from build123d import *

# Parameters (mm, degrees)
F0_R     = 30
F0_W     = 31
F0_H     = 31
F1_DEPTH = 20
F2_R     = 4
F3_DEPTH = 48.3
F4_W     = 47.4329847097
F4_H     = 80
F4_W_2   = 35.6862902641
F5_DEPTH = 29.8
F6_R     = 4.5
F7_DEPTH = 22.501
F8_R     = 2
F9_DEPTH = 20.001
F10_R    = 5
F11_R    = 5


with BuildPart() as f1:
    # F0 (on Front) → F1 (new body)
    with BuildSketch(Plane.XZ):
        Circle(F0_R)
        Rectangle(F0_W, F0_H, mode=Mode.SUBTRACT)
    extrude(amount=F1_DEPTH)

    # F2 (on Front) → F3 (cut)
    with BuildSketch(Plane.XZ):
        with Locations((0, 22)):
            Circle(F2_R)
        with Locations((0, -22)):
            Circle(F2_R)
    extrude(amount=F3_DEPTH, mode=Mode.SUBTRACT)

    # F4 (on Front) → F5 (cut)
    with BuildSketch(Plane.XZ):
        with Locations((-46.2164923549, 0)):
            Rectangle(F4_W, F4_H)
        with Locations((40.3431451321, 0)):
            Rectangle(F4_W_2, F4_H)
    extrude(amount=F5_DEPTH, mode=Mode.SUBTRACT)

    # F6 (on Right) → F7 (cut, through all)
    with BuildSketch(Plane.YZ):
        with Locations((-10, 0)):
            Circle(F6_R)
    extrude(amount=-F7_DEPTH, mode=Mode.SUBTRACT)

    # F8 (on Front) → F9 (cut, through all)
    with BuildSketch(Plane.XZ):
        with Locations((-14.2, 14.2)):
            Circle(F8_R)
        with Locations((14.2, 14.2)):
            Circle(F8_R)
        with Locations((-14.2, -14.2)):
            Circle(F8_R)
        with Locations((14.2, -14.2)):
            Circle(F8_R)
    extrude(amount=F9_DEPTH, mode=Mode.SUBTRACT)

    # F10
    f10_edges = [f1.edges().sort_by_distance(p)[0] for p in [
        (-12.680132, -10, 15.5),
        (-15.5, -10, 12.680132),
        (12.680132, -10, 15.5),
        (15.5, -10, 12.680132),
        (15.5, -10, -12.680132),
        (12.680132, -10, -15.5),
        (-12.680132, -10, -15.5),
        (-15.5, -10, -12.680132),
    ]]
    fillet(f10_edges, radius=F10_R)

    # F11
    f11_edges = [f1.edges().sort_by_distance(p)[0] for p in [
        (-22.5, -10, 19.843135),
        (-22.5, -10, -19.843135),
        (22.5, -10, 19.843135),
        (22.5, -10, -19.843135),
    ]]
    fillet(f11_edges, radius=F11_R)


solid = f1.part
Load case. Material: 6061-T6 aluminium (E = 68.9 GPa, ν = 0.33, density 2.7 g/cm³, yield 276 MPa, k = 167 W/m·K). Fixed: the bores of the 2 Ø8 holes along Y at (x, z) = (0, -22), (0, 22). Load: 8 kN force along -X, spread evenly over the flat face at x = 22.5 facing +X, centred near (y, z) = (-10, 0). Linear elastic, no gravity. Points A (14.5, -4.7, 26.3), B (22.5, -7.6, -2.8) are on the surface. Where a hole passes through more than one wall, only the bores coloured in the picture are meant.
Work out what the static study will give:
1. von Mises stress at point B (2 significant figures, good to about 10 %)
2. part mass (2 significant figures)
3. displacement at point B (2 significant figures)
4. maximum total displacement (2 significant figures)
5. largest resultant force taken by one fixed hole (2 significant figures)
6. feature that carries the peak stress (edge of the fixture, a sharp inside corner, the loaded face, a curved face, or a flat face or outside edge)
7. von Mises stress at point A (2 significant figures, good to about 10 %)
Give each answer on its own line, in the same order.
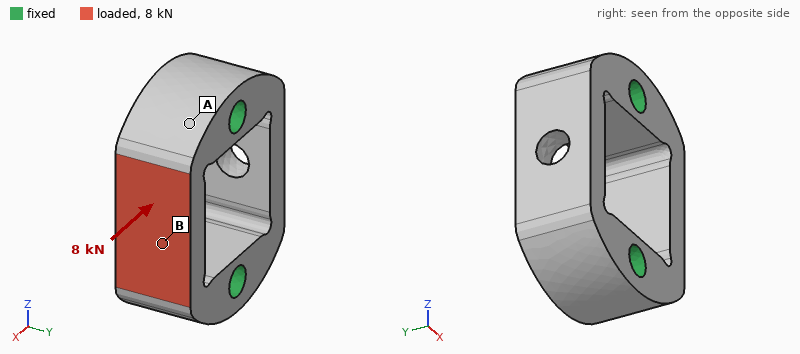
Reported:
100 MPa
71 g
54 µm
61 µm
4.6 kN
a curved face
21 MPa
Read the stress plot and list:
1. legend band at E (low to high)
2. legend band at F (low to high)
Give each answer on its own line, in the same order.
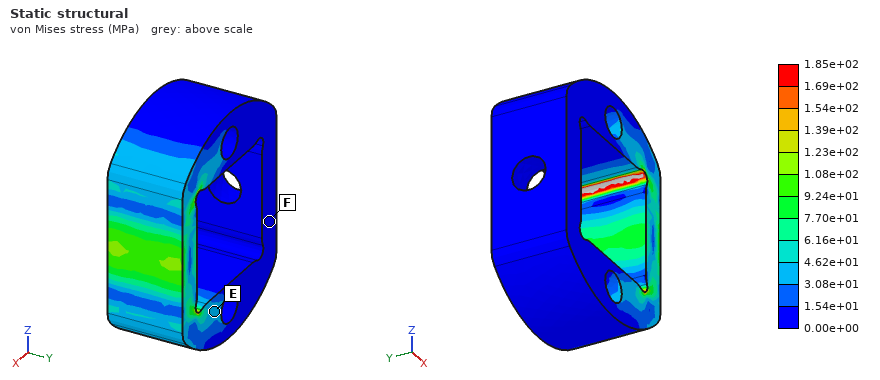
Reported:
3.08e+01 to 4.62e+01 MPa
0.00e+00 to 1.54e+01 MPa
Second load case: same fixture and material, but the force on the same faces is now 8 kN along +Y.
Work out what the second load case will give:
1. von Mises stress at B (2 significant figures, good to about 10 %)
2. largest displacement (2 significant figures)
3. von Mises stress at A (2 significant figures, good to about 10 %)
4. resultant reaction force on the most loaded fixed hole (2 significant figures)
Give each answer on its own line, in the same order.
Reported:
31 MPa
75 µm
23 MPa
4.0 kN
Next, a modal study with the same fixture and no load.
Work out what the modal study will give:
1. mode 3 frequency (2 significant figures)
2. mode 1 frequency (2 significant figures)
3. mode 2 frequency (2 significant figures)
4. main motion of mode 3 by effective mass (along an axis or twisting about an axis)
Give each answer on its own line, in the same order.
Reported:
18 kHz
17 kHz
17 kHz
along Y
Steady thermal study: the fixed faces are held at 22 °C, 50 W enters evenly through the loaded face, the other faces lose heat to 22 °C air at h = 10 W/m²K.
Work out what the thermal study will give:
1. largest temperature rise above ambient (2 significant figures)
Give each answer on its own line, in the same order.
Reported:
22 K
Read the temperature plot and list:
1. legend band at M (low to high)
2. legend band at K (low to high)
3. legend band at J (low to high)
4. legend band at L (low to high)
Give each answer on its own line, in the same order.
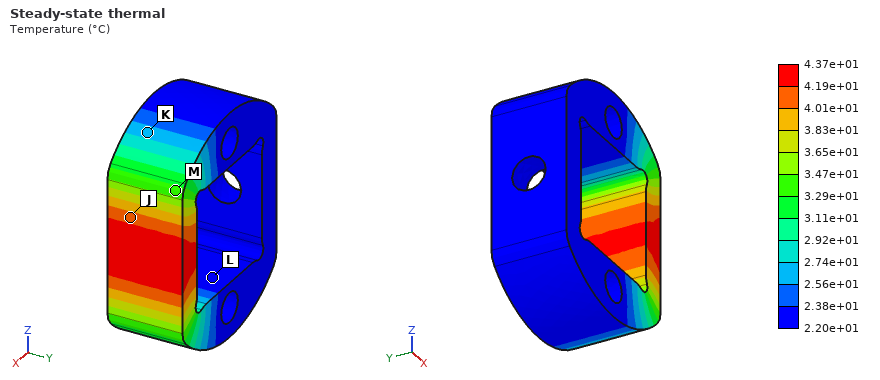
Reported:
3.29e+01 to 3.47e+01 °C
2.56e+01 to 2.74e+01 °C
4.01e+01 to 4.19e+01 °C
2.20e+01 to 2.38e+01 °C
